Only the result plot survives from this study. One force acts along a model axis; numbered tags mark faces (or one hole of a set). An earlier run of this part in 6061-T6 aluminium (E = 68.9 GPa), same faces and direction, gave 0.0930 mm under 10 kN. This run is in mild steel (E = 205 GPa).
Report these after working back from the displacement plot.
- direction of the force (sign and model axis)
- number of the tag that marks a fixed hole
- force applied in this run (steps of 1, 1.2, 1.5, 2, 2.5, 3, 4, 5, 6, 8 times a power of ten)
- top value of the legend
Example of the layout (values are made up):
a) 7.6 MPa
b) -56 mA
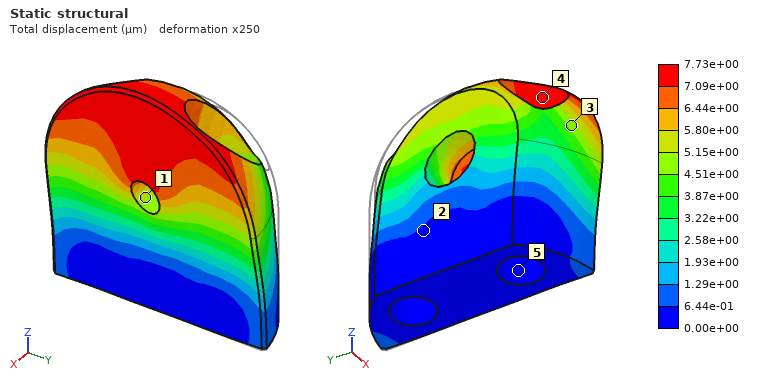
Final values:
a) -Y
b) 5
c) 2.5 kN
d) 7.73e+00 µm
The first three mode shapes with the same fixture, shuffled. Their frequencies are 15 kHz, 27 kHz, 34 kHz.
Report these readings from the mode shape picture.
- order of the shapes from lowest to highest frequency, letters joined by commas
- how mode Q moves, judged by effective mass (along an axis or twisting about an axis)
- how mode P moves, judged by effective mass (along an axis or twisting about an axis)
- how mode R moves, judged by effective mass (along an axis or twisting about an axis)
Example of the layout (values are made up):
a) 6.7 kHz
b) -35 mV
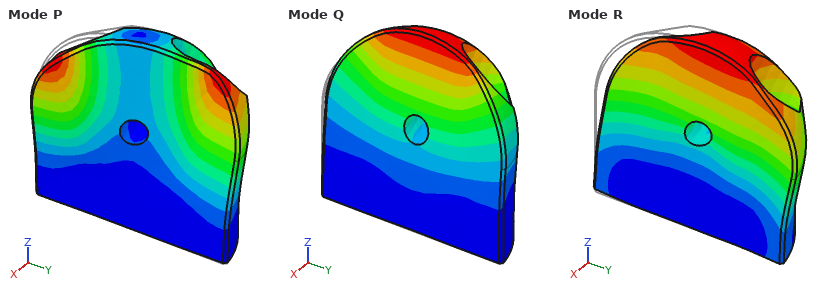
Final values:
a) Q, R, P
b) along X
c) twisting about Z
d) along Y
